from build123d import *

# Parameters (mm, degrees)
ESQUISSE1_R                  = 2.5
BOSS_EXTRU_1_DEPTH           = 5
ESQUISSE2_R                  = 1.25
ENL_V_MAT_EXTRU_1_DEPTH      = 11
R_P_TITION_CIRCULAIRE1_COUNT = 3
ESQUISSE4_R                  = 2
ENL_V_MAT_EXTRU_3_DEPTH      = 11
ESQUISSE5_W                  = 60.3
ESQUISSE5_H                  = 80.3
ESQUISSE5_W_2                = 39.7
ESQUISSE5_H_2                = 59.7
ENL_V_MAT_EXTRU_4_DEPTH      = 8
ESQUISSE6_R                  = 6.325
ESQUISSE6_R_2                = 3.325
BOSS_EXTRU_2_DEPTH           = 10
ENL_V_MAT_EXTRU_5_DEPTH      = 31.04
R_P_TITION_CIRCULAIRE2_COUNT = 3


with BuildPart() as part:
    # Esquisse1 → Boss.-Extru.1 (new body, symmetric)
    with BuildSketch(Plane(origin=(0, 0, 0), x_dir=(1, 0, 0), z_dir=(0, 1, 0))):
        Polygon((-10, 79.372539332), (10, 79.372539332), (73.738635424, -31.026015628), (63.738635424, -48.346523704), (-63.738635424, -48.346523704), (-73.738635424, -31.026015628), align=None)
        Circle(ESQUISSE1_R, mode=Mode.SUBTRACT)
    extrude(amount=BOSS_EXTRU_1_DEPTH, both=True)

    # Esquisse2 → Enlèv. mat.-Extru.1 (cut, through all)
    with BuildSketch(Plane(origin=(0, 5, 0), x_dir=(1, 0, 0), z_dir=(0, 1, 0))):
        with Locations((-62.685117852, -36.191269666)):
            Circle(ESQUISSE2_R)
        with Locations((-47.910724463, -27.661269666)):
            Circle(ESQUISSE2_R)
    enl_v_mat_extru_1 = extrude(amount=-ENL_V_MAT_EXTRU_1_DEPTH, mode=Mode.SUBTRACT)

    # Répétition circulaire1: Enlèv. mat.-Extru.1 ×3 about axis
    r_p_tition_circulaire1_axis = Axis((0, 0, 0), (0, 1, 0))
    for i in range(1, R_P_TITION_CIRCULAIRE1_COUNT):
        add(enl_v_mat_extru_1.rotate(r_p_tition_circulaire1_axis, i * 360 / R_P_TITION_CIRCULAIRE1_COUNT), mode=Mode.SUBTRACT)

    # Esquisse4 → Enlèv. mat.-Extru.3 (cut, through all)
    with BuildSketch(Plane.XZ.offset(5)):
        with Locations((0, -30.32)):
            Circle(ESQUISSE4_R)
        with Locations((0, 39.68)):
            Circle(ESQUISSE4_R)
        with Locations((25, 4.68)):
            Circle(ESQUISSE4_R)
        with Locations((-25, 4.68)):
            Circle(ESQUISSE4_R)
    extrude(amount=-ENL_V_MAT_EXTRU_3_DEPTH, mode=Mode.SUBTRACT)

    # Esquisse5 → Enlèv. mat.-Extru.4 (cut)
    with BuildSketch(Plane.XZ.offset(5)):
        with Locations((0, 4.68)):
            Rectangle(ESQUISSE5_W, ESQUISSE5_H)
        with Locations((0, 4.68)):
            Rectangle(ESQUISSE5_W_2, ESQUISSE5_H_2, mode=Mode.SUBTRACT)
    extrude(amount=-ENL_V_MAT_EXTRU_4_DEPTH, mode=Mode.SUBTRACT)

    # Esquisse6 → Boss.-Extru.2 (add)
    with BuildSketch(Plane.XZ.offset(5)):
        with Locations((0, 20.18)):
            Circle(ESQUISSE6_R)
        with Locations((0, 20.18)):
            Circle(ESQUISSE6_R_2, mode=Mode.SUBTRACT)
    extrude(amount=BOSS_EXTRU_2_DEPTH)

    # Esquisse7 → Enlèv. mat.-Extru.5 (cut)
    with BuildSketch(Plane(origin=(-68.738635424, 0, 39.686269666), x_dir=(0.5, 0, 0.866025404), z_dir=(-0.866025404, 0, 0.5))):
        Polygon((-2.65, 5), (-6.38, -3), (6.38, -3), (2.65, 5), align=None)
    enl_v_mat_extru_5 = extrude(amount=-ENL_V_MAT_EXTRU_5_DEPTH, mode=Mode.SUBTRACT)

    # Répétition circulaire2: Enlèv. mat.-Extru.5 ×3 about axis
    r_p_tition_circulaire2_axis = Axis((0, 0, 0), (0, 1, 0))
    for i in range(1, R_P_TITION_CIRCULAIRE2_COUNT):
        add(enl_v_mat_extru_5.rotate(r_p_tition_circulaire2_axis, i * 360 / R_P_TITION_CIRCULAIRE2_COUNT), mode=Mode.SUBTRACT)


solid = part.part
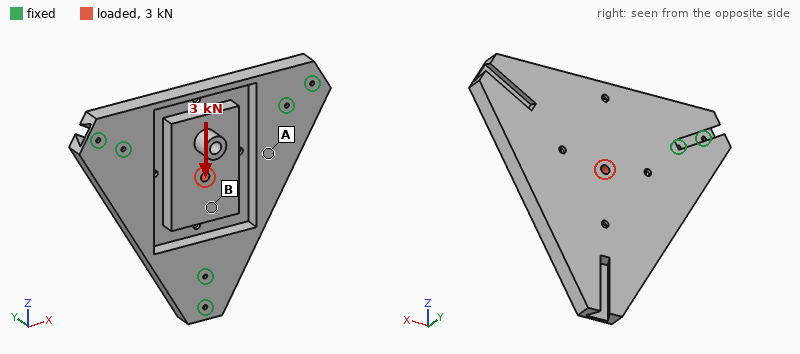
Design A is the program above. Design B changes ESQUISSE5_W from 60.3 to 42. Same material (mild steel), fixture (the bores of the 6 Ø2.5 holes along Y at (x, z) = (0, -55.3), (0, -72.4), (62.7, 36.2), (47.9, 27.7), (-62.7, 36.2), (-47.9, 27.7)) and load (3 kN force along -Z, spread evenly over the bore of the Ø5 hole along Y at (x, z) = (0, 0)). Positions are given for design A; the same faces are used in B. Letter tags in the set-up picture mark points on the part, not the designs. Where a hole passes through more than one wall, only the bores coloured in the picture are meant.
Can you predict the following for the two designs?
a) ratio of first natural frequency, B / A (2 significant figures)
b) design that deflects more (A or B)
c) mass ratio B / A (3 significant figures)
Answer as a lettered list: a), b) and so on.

a) 1.0
b) A
c) 1.13
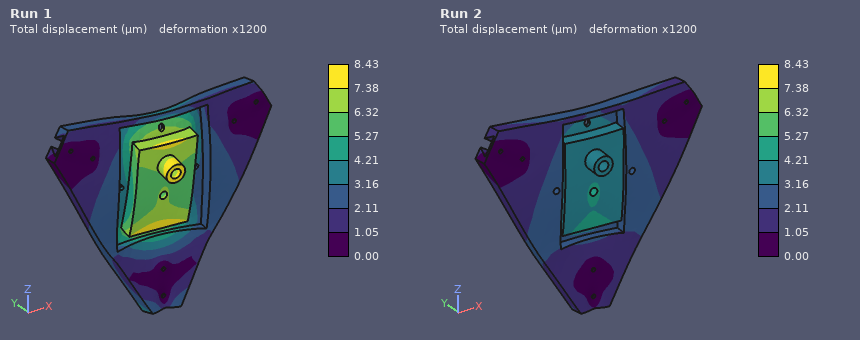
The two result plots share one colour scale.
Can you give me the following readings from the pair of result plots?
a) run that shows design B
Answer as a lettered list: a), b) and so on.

a) Run 2
